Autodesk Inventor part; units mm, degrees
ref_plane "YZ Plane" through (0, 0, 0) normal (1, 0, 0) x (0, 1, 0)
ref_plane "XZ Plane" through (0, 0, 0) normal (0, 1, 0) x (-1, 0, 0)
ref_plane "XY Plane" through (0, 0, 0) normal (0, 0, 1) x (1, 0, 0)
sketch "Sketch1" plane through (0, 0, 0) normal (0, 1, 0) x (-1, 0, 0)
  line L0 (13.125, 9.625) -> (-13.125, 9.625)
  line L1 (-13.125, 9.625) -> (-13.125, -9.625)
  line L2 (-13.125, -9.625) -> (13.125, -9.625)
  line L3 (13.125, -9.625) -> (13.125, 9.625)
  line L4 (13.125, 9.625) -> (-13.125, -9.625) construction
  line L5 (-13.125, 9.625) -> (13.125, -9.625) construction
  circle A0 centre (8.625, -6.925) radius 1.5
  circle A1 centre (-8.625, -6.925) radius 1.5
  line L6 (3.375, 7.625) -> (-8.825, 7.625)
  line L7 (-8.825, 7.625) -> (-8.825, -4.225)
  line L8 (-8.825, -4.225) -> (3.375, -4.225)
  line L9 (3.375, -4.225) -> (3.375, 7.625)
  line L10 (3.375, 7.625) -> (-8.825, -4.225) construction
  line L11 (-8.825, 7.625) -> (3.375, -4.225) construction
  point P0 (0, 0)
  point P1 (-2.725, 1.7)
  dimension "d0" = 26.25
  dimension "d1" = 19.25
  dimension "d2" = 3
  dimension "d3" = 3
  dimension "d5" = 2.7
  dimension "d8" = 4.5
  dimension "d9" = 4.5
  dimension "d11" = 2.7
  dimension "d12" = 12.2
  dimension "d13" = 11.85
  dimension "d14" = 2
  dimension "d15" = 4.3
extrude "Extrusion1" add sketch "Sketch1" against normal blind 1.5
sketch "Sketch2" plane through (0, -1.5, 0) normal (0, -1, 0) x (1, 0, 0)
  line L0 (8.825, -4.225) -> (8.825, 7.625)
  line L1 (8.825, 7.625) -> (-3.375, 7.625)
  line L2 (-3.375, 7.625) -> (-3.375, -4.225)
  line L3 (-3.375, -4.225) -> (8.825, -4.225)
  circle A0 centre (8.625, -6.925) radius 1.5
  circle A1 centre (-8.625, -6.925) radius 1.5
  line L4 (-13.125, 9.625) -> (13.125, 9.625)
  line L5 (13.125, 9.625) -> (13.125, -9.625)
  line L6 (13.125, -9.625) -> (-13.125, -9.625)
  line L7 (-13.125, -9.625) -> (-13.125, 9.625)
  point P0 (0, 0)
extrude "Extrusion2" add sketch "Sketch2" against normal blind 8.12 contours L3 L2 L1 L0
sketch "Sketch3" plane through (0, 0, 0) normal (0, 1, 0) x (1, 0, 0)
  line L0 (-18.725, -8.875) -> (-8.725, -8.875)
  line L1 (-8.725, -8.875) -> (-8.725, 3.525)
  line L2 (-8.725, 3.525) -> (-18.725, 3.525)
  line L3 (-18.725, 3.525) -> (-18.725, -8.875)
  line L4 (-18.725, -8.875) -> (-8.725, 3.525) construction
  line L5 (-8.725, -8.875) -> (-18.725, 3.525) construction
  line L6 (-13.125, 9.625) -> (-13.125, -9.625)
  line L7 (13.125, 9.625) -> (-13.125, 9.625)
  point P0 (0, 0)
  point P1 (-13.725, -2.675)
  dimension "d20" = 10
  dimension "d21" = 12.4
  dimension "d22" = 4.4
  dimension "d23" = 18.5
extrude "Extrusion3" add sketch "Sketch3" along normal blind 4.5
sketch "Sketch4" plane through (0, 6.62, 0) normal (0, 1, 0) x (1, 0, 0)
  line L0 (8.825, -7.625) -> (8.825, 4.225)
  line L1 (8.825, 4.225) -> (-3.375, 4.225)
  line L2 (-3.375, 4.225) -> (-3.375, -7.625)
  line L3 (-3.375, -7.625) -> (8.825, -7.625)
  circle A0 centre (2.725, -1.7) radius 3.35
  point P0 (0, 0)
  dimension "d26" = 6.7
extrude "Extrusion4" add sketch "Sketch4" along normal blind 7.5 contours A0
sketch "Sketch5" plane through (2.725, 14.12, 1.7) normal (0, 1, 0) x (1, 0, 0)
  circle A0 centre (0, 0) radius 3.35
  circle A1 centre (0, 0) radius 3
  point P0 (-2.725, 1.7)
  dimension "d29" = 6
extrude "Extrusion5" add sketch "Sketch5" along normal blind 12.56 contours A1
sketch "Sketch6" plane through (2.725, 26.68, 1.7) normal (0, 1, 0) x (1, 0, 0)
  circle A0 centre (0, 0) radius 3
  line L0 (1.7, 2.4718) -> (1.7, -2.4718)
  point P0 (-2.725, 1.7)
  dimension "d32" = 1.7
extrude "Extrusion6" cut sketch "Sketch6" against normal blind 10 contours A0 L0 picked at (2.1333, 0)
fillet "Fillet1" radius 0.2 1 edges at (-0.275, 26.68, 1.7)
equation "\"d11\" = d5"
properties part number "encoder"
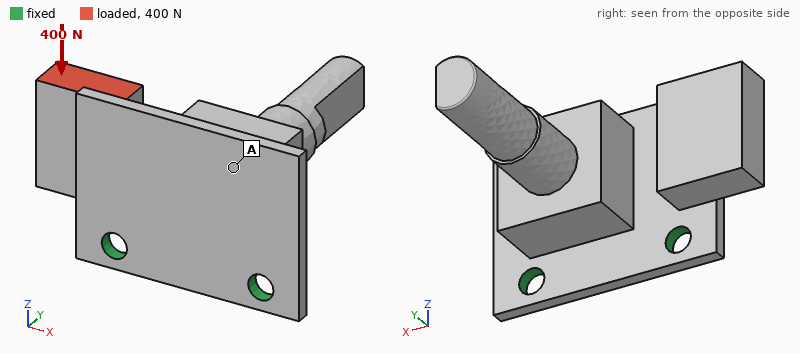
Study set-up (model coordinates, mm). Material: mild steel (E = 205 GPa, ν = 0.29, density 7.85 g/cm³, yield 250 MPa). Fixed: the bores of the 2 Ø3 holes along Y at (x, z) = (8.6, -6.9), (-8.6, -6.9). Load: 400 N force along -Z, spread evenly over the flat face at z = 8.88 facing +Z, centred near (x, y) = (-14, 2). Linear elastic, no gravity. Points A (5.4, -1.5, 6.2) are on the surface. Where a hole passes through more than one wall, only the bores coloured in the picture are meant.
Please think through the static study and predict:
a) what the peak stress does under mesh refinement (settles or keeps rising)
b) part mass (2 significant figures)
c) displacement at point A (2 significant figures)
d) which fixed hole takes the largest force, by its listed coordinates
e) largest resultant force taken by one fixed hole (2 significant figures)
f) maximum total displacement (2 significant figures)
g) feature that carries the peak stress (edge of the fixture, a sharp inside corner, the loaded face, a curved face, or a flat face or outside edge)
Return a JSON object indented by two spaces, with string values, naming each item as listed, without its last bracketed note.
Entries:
{
  "what the peak stress does under mesh refinement": "keeps rising",
  "part mass": "22 g",
  "displacement at point A": "29 µm",
  "which fixed hole takes the largest force, by its listed coordinates": "(-8.6, -6.9)",
  "largest resultant force taken by one fixed hole": "490 N",
  "maximum total displacement": "77 µm",
  "feature that carries the peak stress": "edge of the fixture"
}
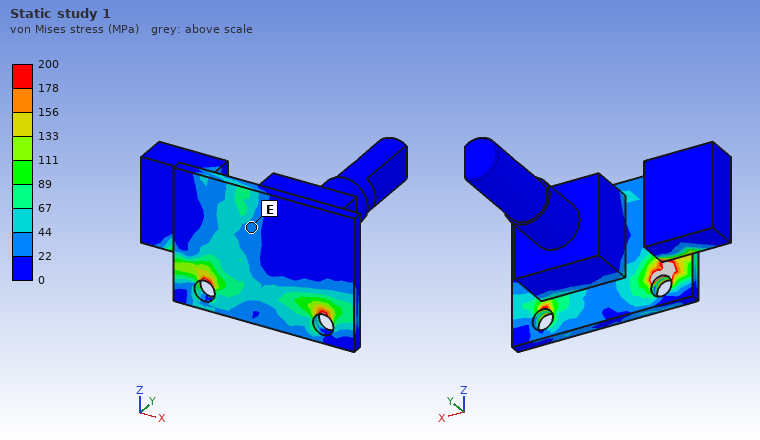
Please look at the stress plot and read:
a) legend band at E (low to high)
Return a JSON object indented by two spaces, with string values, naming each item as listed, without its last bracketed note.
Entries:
{
  "legend band at E": "22 to 44 MPa"
}
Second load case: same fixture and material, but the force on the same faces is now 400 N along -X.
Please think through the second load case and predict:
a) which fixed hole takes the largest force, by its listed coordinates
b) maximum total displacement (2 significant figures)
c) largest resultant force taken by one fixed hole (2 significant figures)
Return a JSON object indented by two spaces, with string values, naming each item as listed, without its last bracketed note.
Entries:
{
  "which fixed hole takes the largest force, by its listed coordinates": "(8.6, -6.9)",
  "maximum total displacement": "49 µm",
  "largest resultant force taken by one fixed hole": "410 N"
}
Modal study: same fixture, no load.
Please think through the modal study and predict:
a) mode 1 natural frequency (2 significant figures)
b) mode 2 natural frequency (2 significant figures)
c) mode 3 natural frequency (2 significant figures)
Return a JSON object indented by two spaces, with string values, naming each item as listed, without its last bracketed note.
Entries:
{
  "mode 1 natural frequency": "1900 Hz",
  "mode 2 natural frequency": "5000 Hz",
  "mode 3 natural frequency": "6100 Hz"
}
